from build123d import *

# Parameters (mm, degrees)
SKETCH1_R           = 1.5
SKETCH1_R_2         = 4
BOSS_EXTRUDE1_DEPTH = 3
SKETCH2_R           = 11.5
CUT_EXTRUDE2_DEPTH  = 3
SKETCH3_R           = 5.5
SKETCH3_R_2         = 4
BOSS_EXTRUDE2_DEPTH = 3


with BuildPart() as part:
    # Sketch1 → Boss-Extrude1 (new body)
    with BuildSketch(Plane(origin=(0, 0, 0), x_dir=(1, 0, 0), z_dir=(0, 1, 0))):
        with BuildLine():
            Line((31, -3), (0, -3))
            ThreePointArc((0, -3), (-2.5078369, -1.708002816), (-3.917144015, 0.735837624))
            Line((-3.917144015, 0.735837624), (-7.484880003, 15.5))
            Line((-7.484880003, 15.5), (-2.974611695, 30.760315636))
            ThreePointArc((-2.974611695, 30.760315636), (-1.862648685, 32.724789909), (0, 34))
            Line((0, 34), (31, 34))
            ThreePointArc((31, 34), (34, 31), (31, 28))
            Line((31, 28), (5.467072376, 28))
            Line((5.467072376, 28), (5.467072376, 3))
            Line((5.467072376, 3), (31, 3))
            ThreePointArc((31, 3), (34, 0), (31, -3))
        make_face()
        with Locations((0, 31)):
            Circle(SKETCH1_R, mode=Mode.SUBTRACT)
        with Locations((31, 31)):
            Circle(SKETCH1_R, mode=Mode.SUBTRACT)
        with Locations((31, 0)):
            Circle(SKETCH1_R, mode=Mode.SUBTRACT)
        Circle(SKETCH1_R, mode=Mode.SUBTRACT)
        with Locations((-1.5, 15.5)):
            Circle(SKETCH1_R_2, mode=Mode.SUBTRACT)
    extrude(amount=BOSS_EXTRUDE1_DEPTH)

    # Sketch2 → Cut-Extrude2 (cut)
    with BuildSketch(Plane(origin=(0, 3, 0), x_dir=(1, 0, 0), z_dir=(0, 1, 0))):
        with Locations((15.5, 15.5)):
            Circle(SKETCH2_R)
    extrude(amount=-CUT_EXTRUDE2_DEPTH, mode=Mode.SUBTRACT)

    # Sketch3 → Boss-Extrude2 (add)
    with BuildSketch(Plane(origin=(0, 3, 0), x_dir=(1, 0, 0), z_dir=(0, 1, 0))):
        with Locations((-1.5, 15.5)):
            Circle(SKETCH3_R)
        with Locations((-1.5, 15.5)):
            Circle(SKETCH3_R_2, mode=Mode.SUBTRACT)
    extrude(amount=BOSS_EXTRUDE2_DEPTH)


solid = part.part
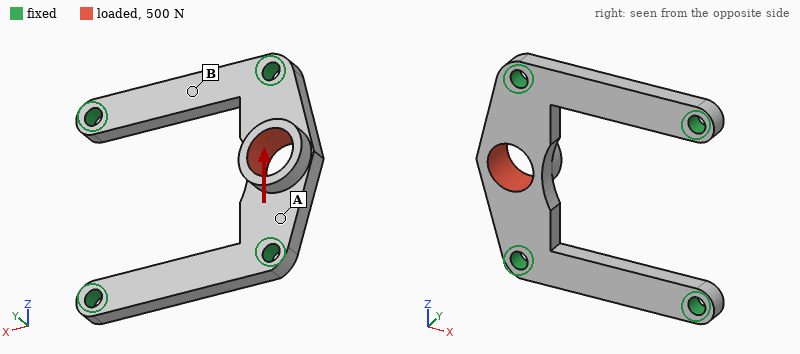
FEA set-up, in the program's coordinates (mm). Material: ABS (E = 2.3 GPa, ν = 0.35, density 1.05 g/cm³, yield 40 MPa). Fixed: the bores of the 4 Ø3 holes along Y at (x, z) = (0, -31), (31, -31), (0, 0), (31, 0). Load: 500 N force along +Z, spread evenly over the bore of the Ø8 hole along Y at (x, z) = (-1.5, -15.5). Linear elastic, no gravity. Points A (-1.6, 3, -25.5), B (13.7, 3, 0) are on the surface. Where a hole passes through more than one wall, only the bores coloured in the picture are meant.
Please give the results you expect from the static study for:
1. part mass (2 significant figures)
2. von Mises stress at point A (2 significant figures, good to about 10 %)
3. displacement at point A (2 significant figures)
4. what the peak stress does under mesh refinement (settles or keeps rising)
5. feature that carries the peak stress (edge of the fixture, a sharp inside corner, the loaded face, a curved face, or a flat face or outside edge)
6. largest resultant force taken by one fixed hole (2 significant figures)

2.1 g
14 MPa
0.036 mm
keeps rising
edge of the fixture
260 N
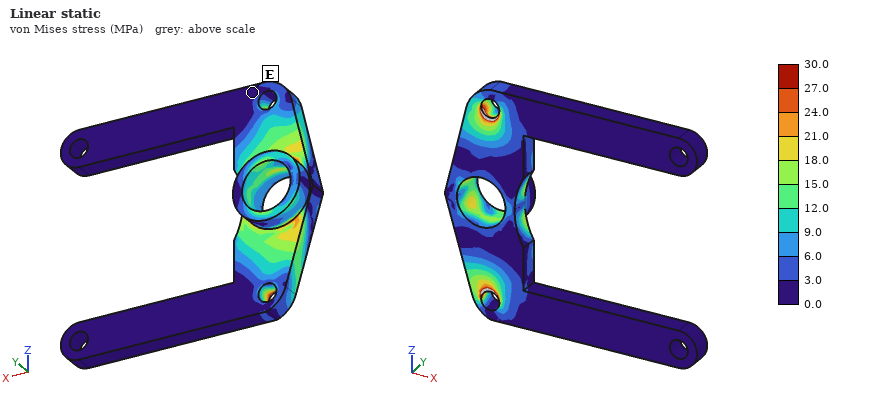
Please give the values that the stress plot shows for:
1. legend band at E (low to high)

0.0 to 3.0 MPa
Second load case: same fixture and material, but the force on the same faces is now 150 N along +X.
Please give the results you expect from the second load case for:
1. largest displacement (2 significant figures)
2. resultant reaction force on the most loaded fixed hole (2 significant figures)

0.23 mm
69 N
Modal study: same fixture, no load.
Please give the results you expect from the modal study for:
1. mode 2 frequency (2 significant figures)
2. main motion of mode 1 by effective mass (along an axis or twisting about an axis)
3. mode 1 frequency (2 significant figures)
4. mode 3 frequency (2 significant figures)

5100 Hz
along Y
4500 Hz
5200 Hz
